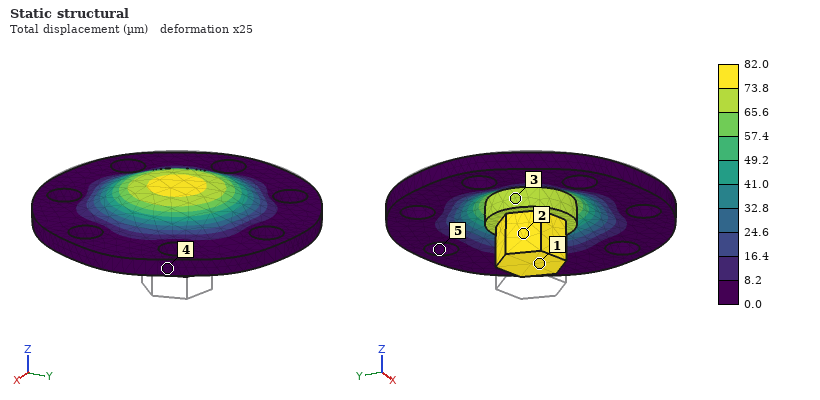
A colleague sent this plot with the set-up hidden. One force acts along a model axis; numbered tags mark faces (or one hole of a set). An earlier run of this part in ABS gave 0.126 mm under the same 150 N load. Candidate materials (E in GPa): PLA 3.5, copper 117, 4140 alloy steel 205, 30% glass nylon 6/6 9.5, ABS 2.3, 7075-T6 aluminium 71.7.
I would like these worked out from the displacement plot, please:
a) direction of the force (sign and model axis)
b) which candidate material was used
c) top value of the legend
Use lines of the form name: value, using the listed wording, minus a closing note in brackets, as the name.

direction of the force: +Z
which candidate material was used: PLA
top value of the legend: 82.0 µm
